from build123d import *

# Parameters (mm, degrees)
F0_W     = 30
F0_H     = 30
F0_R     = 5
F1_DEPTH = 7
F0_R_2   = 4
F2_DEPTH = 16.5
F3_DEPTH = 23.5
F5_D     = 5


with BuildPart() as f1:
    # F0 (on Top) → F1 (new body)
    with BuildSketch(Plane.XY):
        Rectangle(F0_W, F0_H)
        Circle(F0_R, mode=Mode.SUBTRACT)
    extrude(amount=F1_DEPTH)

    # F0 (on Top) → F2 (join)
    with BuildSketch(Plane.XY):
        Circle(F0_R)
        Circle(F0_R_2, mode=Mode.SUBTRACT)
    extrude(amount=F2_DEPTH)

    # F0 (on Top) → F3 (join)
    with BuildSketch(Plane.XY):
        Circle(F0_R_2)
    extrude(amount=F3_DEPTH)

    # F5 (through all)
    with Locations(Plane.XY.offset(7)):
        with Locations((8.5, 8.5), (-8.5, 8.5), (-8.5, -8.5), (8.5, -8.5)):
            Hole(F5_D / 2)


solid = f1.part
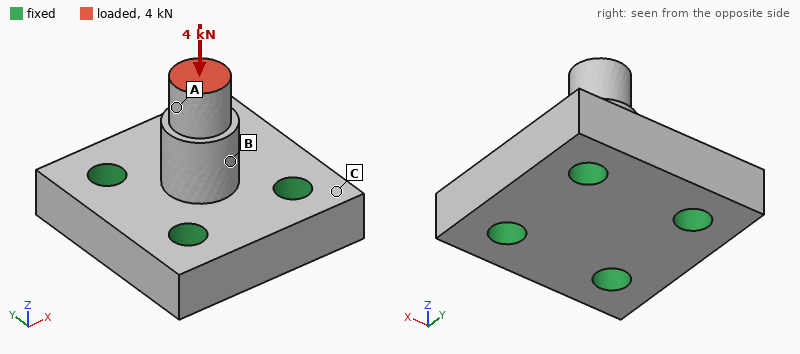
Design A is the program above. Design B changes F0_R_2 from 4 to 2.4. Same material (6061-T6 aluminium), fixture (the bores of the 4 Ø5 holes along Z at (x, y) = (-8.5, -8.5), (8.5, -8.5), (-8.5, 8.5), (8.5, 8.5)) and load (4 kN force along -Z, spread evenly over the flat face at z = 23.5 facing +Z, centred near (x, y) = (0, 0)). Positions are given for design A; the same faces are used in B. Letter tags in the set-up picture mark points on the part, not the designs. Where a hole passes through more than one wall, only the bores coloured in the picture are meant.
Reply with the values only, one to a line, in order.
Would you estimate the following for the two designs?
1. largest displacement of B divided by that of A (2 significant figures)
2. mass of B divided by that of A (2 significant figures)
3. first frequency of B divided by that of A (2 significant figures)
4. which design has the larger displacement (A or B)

1.8
0.97
1.3
B
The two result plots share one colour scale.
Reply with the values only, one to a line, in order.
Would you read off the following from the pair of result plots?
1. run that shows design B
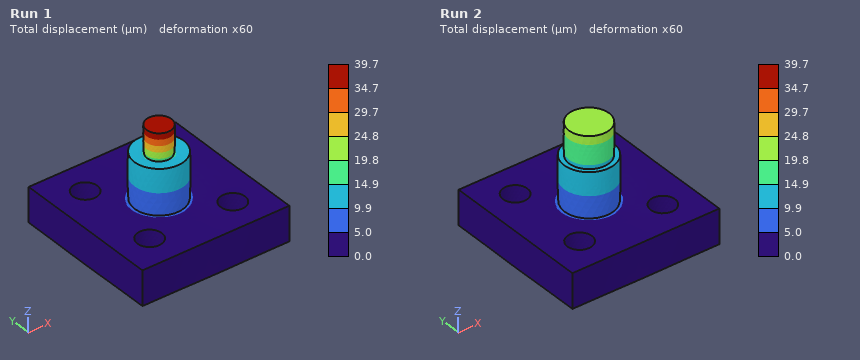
Run 1
